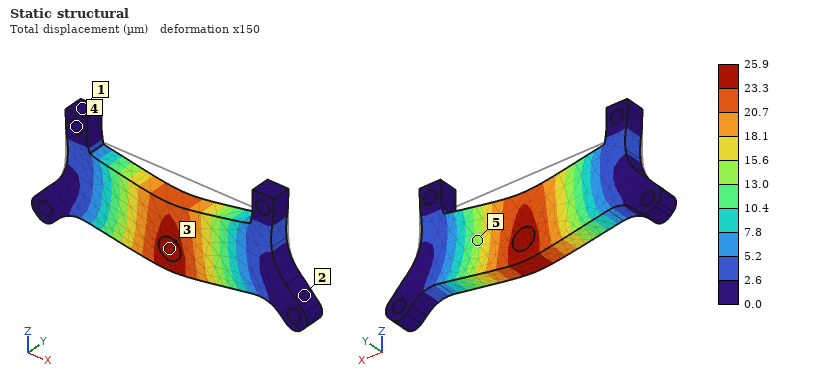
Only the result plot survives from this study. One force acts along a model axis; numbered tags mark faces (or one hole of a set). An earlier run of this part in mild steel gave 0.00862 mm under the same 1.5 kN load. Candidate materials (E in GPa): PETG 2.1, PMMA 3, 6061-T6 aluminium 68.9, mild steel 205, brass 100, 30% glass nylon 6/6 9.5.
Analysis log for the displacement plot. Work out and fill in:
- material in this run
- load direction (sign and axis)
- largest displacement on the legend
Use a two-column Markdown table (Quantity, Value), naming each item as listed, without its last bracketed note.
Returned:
| Quantity | Value |
|---|---|
| material in this run | 6061-T6 aluminium |
| load direction | -Z |
| largest displacement on the legend | 25.9 µm |
